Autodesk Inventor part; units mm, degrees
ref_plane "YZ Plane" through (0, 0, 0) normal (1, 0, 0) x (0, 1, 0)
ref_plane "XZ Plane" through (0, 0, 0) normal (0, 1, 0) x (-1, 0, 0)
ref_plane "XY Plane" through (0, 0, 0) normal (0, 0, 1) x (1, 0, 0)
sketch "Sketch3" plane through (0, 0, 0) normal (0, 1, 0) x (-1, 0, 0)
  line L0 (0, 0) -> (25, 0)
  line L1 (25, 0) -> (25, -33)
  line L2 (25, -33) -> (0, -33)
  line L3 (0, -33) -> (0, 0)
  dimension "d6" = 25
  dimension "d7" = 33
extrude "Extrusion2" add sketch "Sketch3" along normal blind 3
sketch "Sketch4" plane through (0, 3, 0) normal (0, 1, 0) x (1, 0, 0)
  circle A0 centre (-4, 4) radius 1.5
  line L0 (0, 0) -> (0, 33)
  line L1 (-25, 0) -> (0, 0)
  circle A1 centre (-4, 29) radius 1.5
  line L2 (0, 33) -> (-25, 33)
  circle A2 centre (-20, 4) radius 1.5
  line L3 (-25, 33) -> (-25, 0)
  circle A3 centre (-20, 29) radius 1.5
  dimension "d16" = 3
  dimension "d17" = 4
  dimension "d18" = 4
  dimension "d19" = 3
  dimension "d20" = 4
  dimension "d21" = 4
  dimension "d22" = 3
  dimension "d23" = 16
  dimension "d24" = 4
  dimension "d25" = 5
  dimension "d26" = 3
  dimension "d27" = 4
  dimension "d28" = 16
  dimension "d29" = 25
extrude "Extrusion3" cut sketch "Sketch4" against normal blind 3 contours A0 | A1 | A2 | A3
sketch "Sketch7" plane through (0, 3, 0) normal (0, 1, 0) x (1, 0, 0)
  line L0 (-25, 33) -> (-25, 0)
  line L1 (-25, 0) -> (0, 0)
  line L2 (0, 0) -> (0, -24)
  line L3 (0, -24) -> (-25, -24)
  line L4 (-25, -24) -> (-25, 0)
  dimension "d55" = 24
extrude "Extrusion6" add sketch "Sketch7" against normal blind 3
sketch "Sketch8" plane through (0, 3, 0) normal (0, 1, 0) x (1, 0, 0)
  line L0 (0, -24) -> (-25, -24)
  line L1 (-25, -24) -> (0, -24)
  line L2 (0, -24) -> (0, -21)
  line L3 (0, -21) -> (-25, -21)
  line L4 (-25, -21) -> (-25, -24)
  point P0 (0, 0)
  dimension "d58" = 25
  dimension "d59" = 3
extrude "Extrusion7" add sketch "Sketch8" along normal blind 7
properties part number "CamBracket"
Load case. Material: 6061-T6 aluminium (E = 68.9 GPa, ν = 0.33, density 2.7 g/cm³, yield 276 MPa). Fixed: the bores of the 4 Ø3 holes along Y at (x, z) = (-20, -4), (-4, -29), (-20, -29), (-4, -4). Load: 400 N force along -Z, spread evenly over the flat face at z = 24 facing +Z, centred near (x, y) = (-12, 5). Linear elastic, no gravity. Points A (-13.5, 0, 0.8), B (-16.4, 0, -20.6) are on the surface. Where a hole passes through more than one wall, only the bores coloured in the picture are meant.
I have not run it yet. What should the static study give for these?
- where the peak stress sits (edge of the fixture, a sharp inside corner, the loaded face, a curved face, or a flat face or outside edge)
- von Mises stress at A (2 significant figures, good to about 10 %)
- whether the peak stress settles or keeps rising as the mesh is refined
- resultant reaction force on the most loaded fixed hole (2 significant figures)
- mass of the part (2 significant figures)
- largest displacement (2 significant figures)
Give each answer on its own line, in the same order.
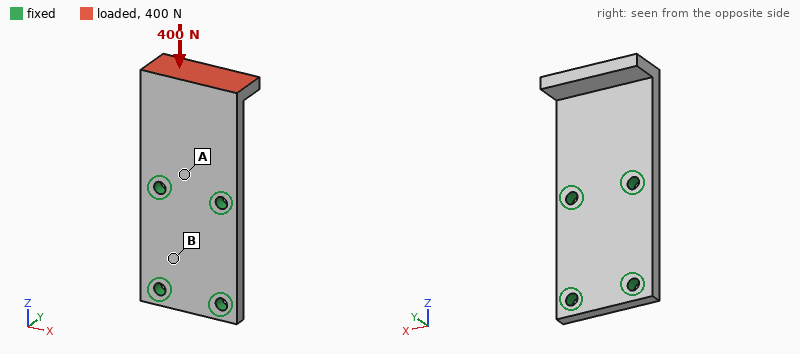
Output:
edge of the fixture
28 MPa
keeps rising
190 N
13 g
0.16 mm
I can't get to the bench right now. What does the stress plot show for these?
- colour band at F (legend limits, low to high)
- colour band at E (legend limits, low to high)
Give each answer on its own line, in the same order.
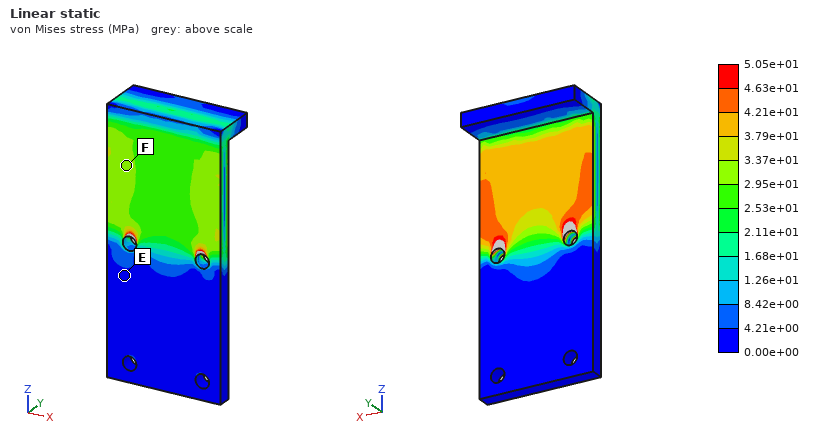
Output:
2.95e+01 to 3.37e+01 MPa
0.00e+00 to 4.21e+00 MPa
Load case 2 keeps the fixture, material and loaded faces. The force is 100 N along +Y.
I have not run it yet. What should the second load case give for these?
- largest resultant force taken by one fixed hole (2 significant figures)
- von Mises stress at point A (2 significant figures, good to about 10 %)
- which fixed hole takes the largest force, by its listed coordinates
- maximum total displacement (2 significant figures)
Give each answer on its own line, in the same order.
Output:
61 N
50 MPa
(-20, -4)
0.20 mm
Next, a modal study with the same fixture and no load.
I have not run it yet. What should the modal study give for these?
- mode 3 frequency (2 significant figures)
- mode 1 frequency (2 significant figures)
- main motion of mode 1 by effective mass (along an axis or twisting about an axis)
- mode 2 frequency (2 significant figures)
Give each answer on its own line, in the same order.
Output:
13 kHz
2300 Hz
along Y
5900 Hz
